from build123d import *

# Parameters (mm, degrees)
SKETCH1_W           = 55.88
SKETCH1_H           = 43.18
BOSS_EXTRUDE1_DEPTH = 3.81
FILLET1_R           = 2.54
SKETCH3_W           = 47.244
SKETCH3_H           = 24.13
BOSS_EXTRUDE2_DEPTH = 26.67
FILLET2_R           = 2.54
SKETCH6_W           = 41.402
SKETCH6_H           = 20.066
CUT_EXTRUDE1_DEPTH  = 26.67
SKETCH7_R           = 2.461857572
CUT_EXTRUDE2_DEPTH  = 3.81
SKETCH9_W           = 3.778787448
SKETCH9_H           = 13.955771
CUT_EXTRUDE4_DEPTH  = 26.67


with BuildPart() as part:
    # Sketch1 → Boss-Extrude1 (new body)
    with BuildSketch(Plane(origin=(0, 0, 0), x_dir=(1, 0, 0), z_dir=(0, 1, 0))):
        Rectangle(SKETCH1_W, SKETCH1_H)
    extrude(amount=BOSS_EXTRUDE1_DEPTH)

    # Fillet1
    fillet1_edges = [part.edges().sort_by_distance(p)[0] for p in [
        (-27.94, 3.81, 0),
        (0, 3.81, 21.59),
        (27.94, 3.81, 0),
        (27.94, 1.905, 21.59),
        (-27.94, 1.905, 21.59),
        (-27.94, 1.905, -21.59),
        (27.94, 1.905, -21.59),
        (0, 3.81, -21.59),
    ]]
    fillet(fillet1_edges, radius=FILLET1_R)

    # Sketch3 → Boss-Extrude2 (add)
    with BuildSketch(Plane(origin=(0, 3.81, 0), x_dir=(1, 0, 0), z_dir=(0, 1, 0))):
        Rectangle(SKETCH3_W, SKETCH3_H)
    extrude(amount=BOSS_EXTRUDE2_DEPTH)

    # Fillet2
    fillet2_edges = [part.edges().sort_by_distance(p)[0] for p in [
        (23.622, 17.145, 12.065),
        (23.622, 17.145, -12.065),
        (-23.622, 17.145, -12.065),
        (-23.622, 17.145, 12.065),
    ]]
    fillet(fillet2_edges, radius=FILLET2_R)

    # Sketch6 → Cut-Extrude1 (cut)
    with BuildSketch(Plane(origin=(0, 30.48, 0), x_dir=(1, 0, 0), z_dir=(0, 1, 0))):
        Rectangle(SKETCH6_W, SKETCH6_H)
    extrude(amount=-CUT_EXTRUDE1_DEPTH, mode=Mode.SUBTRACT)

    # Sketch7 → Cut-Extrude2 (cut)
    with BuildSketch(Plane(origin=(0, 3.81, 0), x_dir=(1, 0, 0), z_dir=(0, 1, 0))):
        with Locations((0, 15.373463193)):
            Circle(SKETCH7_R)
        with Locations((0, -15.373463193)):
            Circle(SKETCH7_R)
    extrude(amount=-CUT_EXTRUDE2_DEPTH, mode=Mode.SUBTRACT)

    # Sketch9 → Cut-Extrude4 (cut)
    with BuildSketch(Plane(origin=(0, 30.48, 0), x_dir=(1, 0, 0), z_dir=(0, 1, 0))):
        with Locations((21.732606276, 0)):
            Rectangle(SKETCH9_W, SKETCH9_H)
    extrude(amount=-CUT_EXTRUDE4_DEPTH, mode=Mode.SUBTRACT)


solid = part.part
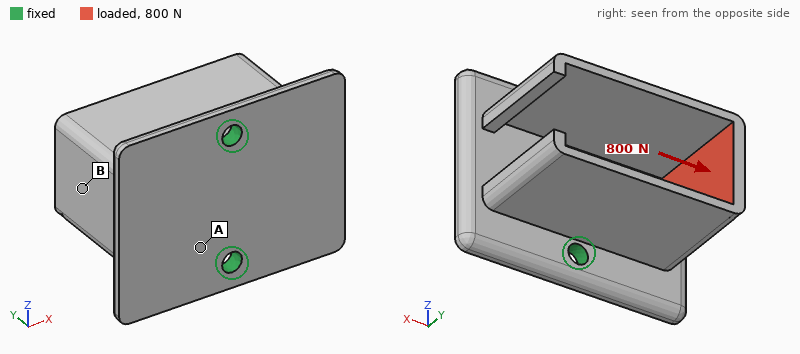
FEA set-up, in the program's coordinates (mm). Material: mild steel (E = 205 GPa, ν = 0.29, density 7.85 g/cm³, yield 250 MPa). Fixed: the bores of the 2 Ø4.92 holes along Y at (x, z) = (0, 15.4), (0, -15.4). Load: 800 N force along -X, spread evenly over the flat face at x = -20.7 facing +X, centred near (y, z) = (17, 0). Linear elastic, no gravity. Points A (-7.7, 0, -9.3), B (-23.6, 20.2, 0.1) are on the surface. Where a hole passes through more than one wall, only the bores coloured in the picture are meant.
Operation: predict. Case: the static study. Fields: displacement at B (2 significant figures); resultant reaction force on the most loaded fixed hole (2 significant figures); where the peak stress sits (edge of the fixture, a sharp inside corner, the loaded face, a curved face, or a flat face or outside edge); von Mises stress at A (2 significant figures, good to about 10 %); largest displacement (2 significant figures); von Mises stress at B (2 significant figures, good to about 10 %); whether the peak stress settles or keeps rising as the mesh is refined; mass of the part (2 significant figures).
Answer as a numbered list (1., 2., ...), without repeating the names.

1. 27 µm
2. 400 N
3. edge of the fixture
4. 14 MPa
5. 36 µm
6. 34 MPa
7. keeps rising
8. 120 g
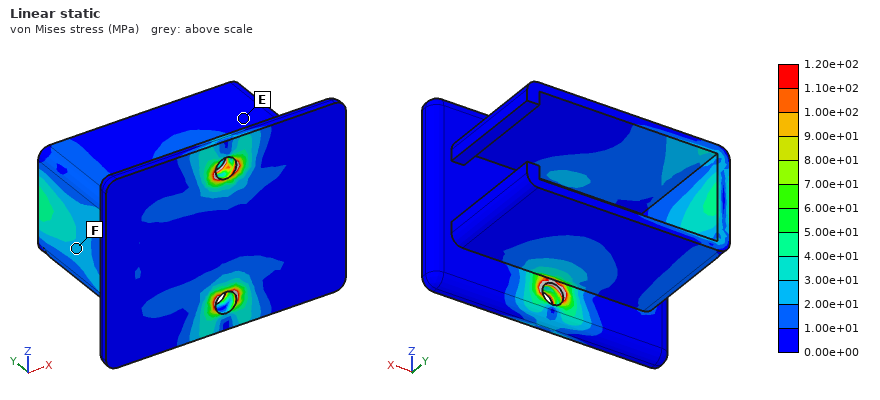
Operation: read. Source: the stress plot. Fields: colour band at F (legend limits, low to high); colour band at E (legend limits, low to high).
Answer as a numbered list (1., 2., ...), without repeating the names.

1. 2.00e+01 to 3.00e+01 MPa
2. 0.00e+00 to 1.00e+01 MPa
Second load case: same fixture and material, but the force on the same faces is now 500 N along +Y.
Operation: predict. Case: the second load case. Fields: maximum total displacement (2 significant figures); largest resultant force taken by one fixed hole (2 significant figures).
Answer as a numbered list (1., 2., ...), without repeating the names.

1. 24 µm
2. 250 N
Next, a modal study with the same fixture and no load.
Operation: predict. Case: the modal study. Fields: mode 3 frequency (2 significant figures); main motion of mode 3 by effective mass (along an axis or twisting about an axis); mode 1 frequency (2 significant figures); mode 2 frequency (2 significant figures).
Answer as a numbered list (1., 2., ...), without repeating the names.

1. 4000 Hz
2. along Z
3. 3000 Hz
4. 3600 Hz
